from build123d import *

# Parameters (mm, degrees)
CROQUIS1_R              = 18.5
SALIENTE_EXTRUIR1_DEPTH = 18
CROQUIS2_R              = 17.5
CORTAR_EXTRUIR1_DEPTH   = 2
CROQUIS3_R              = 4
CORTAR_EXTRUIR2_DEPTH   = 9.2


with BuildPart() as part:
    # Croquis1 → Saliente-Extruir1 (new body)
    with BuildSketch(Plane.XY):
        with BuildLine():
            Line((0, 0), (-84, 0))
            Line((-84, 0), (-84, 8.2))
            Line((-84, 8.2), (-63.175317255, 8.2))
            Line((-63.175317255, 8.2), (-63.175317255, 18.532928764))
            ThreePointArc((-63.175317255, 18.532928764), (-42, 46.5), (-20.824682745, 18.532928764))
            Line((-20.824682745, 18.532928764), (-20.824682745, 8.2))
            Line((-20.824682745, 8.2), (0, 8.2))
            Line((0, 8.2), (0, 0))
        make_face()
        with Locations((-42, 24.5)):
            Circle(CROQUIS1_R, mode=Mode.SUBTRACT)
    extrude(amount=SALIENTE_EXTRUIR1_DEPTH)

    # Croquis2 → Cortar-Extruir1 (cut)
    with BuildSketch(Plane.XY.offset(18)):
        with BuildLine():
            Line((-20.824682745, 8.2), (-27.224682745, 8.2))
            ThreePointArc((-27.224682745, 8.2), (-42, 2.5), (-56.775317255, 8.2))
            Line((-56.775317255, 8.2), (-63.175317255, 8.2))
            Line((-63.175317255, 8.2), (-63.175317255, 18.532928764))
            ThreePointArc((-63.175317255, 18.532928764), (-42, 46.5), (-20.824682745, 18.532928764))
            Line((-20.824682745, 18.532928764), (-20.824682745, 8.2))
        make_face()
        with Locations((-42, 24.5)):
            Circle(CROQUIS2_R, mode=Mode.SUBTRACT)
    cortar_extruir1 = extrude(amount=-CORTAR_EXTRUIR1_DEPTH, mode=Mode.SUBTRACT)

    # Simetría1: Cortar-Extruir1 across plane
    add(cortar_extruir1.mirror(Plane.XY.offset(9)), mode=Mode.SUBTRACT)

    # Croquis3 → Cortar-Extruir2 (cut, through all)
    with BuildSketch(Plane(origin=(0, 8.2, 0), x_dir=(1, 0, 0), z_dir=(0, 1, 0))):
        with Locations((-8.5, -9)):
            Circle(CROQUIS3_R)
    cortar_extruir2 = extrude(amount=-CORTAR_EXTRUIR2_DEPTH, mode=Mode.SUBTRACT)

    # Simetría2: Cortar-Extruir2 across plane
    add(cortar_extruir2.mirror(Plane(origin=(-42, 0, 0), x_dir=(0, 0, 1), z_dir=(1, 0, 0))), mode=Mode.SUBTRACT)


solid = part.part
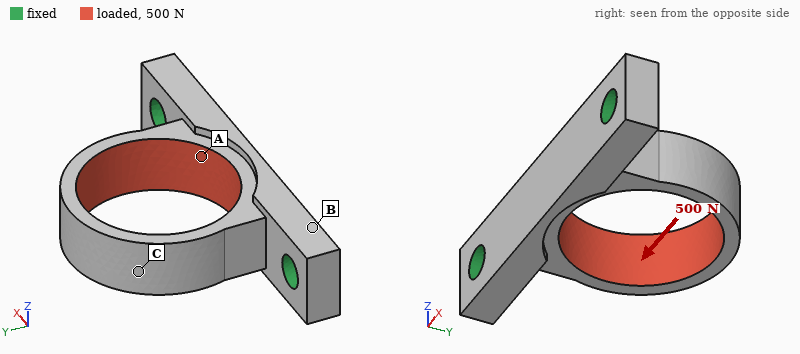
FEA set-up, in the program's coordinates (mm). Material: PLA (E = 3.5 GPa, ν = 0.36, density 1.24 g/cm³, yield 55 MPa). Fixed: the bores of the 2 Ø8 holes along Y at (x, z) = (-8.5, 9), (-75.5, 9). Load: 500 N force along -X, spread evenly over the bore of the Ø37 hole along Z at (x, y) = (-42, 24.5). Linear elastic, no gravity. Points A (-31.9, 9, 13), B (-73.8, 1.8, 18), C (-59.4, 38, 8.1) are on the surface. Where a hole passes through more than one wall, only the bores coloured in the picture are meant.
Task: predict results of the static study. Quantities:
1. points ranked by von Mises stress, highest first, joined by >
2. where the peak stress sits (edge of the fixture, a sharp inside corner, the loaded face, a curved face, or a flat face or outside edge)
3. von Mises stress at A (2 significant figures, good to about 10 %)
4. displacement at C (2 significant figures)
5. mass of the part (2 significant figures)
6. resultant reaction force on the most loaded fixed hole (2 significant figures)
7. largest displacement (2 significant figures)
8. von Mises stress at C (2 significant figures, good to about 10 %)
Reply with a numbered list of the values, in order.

1. C > A > B
2. a curved face
3. 8.2 MPa
4. 1.1 mm
5. 20 g
6. 310 N
7. 1.1 mm
8. 19 MPa
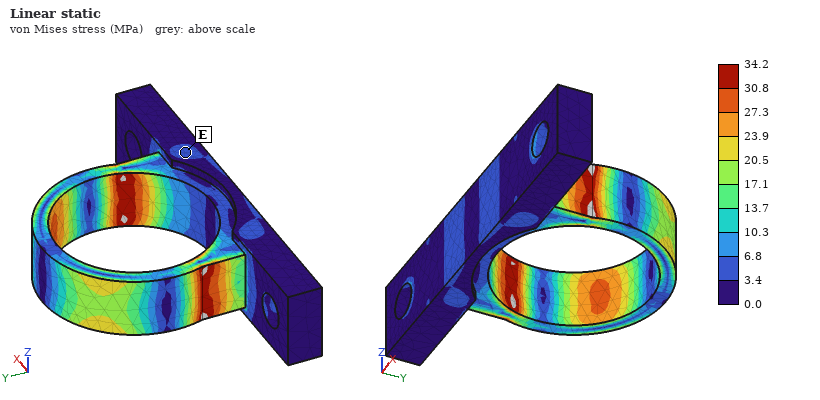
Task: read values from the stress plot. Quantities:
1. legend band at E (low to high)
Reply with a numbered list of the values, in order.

1. 3.4 to 6.8 MPa
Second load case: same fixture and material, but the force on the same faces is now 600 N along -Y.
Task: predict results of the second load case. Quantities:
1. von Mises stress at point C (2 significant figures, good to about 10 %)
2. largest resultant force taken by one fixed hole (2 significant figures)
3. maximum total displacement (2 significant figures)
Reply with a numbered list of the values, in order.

1. 2.3 MPa
2. 300 N
3. 0.20 mm
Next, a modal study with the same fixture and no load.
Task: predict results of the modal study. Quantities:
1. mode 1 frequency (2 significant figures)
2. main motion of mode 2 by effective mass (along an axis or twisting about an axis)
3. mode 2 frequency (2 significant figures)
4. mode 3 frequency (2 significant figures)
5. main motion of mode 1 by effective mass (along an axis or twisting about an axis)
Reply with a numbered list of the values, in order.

1. 1200 Hz
2. along X
3. 1300 Hz
4. 2700 Hz
5. along Z
